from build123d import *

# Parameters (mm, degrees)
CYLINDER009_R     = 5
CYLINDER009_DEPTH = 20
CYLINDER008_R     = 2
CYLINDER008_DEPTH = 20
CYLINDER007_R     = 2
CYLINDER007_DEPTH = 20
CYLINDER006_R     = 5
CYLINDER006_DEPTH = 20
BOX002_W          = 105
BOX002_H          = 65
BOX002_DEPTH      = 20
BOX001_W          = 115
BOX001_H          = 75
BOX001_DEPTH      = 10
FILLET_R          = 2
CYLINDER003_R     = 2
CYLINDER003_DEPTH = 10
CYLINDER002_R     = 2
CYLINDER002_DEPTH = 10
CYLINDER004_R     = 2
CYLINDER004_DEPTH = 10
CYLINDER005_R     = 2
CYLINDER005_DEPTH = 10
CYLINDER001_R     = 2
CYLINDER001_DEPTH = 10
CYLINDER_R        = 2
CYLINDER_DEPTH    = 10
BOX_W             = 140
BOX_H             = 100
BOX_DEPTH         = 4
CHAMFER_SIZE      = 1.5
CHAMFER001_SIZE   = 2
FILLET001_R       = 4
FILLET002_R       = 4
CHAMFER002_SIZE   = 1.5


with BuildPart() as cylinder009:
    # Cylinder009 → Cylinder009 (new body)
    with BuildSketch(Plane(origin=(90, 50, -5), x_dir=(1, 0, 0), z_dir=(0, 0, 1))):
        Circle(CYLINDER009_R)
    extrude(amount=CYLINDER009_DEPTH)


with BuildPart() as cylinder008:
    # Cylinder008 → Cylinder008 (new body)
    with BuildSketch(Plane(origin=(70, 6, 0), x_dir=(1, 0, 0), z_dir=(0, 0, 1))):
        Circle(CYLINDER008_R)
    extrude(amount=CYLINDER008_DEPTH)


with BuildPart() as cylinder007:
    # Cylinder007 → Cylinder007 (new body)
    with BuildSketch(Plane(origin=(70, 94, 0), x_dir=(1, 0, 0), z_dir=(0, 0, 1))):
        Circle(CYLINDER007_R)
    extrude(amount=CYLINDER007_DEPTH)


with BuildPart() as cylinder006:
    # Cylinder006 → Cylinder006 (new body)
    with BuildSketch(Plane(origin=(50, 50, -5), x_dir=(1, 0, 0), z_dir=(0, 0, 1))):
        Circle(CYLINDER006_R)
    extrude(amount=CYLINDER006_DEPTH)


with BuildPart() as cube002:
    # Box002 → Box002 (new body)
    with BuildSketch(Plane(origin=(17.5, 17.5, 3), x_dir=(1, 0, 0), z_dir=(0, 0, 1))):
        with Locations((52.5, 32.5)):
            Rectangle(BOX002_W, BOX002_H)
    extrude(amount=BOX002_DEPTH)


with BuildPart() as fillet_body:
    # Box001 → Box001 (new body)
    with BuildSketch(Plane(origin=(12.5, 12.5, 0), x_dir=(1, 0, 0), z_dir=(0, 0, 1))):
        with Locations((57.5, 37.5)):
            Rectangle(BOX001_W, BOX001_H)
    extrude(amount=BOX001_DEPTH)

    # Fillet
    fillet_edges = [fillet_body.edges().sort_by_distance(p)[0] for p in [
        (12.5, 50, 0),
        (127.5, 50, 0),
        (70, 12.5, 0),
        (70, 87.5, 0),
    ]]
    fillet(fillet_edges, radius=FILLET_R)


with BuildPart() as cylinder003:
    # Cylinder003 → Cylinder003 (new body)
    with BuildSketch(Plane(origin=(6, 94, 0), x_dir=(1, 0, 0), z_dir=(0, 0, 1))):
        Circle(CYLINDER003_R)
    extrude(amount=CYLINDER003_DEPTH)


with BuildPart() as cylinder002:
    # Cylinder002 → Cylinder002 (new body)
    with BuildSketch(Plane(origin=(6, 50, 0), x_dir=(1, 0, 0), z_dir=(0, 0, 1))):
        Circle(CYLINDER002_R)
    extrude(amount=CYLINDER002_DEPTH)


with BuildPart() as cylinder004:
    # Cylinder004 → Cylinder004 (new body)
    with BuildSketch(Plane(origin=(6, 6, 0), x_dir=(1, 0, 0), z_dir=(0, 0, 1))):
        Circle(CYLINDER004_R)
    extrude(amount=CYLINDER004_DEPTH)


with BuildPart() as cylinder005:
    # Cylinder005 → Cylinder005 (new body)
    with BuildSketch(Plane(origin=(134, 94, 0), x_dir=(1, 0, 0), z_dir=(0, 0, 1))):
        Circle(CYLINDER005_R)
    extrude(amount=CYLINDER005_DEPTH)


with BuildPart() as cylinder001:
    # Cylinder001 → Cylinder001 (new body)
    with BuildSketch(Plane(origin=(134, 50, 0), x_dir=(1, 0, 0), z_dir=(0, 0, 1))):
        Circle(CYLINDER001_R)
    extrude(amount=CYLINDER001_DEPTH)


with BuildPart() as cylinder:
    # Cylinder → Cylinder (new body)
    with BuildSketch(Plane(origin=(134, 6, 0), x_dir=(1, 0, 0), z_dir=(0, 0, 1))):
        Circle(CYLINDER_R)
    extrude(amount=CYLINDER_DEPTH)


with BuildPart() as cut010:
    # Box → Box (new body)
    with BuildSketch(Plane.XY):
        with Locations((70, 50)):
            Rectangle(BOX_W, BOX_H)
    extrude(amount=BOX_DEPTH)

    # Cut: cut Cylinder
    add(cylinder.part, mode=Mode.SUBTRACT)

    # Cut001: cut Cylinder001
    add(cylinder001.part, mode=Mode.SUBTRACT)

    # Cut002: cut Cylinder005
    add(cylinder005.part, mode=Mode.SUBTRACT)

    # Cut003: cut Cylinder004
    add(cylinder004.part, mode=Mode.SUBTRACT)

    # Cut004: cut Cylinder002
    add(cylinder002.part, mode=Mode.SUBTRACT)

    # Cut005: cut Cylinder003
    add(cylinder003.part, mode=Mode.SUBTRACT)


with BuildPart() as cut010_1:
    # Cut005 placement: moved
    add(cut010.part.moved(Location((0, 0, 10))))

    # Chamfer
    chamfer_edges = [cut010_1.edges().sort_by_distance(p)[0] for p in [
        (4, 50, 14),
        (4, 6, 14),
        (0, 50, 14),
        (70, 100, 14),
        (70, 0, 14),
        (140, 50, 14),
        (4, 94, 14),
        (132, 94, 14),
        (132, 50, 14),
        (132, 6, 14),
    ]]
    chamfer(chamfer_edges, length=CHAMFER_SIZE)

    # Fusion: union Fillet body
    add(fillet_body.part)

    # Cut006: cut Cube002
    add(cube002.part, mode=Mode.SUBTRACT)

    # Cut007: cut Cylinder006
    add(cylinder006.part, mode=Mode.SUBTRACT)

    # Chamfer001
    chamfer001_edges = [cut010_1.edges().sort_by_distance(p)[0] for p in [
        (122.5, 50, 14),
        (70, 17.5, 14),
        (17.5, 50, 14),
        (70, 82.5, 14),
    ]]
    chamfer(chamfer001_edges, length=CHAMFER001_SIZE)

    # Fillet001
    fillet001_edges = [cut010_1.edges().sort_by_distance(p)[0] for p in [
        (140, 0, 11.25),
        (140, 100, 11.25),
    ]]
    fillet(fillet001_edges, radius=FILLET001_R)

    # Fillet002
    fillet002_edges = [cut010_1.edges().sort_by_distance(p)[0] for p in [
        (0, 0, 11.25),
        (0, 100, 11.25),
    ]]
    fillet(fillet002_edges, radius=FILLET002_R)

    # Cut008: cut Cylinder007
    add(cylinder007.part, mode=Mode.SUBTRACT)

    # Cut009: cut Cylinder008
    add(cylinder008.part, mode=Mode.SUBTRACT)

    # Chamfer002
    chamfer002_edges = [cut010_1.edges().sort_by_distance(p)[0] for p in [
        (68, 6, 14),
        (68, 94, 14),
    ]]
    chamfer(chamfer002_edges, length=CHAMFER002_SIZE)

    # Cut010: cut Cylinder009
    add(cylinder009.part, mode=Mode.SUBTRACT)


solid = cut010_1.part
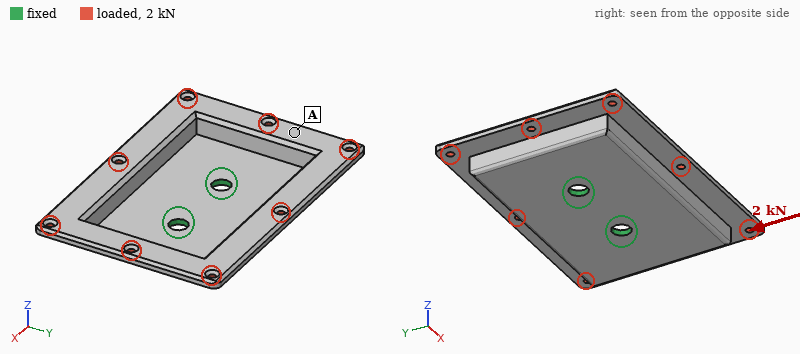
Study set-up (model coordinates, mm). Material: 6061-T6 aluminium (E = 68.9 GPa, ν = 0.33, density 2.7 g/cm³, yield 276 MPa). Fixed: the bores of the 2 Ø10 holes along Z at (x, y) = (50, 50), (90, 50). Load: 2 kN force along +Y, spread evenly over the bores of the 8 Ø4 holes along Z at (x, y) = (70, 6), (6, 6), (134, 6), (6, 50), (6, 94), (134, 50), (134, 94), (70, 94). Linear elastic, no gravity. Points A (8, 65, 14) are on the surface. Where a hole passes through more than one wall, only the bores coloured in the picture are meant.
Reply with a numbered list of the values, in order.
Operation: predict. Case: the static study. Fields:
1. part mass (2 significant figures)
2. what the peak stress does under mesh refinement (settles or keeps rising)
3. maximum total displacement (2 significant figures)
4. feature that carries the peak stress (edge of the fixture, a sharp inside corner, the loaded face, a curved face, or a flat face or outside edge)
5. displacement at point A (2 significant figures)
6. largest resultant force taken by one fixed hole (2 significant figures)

1. 170 g
2. keeps rising
3. 0.38 mm
4. edge of the fixture
5. 0.15 mm
6. 1.0 kN
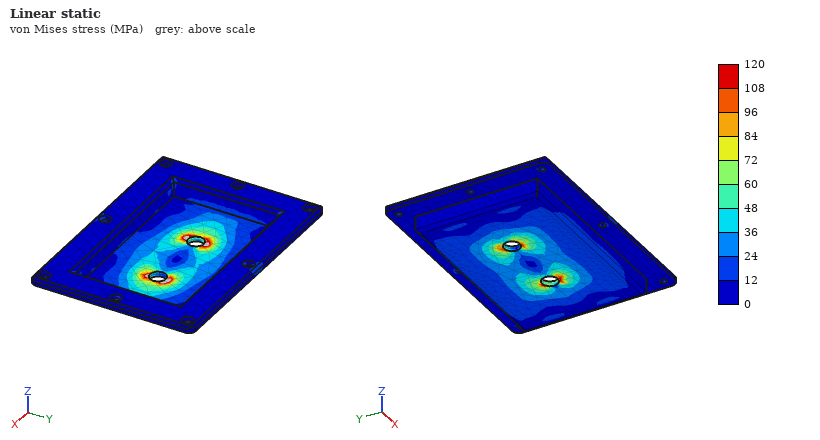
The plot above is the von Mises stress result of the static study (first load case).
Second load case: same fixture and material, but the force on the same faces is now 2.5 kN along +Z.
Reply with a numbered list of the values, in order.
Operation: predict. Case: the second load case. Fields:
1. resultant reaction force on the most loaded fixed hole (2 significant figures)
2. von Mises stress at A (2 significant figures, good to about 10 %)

1. 1.6 kN
2. 28 MPa
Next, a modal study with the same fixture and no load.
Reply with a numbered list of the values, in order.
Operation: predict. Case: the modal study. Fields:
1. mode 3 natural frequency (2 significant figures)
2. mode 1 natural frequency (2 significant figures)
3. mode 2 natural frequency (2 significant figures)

1. 1100 Hz
2. 710 Hz
3. 940 Hz
